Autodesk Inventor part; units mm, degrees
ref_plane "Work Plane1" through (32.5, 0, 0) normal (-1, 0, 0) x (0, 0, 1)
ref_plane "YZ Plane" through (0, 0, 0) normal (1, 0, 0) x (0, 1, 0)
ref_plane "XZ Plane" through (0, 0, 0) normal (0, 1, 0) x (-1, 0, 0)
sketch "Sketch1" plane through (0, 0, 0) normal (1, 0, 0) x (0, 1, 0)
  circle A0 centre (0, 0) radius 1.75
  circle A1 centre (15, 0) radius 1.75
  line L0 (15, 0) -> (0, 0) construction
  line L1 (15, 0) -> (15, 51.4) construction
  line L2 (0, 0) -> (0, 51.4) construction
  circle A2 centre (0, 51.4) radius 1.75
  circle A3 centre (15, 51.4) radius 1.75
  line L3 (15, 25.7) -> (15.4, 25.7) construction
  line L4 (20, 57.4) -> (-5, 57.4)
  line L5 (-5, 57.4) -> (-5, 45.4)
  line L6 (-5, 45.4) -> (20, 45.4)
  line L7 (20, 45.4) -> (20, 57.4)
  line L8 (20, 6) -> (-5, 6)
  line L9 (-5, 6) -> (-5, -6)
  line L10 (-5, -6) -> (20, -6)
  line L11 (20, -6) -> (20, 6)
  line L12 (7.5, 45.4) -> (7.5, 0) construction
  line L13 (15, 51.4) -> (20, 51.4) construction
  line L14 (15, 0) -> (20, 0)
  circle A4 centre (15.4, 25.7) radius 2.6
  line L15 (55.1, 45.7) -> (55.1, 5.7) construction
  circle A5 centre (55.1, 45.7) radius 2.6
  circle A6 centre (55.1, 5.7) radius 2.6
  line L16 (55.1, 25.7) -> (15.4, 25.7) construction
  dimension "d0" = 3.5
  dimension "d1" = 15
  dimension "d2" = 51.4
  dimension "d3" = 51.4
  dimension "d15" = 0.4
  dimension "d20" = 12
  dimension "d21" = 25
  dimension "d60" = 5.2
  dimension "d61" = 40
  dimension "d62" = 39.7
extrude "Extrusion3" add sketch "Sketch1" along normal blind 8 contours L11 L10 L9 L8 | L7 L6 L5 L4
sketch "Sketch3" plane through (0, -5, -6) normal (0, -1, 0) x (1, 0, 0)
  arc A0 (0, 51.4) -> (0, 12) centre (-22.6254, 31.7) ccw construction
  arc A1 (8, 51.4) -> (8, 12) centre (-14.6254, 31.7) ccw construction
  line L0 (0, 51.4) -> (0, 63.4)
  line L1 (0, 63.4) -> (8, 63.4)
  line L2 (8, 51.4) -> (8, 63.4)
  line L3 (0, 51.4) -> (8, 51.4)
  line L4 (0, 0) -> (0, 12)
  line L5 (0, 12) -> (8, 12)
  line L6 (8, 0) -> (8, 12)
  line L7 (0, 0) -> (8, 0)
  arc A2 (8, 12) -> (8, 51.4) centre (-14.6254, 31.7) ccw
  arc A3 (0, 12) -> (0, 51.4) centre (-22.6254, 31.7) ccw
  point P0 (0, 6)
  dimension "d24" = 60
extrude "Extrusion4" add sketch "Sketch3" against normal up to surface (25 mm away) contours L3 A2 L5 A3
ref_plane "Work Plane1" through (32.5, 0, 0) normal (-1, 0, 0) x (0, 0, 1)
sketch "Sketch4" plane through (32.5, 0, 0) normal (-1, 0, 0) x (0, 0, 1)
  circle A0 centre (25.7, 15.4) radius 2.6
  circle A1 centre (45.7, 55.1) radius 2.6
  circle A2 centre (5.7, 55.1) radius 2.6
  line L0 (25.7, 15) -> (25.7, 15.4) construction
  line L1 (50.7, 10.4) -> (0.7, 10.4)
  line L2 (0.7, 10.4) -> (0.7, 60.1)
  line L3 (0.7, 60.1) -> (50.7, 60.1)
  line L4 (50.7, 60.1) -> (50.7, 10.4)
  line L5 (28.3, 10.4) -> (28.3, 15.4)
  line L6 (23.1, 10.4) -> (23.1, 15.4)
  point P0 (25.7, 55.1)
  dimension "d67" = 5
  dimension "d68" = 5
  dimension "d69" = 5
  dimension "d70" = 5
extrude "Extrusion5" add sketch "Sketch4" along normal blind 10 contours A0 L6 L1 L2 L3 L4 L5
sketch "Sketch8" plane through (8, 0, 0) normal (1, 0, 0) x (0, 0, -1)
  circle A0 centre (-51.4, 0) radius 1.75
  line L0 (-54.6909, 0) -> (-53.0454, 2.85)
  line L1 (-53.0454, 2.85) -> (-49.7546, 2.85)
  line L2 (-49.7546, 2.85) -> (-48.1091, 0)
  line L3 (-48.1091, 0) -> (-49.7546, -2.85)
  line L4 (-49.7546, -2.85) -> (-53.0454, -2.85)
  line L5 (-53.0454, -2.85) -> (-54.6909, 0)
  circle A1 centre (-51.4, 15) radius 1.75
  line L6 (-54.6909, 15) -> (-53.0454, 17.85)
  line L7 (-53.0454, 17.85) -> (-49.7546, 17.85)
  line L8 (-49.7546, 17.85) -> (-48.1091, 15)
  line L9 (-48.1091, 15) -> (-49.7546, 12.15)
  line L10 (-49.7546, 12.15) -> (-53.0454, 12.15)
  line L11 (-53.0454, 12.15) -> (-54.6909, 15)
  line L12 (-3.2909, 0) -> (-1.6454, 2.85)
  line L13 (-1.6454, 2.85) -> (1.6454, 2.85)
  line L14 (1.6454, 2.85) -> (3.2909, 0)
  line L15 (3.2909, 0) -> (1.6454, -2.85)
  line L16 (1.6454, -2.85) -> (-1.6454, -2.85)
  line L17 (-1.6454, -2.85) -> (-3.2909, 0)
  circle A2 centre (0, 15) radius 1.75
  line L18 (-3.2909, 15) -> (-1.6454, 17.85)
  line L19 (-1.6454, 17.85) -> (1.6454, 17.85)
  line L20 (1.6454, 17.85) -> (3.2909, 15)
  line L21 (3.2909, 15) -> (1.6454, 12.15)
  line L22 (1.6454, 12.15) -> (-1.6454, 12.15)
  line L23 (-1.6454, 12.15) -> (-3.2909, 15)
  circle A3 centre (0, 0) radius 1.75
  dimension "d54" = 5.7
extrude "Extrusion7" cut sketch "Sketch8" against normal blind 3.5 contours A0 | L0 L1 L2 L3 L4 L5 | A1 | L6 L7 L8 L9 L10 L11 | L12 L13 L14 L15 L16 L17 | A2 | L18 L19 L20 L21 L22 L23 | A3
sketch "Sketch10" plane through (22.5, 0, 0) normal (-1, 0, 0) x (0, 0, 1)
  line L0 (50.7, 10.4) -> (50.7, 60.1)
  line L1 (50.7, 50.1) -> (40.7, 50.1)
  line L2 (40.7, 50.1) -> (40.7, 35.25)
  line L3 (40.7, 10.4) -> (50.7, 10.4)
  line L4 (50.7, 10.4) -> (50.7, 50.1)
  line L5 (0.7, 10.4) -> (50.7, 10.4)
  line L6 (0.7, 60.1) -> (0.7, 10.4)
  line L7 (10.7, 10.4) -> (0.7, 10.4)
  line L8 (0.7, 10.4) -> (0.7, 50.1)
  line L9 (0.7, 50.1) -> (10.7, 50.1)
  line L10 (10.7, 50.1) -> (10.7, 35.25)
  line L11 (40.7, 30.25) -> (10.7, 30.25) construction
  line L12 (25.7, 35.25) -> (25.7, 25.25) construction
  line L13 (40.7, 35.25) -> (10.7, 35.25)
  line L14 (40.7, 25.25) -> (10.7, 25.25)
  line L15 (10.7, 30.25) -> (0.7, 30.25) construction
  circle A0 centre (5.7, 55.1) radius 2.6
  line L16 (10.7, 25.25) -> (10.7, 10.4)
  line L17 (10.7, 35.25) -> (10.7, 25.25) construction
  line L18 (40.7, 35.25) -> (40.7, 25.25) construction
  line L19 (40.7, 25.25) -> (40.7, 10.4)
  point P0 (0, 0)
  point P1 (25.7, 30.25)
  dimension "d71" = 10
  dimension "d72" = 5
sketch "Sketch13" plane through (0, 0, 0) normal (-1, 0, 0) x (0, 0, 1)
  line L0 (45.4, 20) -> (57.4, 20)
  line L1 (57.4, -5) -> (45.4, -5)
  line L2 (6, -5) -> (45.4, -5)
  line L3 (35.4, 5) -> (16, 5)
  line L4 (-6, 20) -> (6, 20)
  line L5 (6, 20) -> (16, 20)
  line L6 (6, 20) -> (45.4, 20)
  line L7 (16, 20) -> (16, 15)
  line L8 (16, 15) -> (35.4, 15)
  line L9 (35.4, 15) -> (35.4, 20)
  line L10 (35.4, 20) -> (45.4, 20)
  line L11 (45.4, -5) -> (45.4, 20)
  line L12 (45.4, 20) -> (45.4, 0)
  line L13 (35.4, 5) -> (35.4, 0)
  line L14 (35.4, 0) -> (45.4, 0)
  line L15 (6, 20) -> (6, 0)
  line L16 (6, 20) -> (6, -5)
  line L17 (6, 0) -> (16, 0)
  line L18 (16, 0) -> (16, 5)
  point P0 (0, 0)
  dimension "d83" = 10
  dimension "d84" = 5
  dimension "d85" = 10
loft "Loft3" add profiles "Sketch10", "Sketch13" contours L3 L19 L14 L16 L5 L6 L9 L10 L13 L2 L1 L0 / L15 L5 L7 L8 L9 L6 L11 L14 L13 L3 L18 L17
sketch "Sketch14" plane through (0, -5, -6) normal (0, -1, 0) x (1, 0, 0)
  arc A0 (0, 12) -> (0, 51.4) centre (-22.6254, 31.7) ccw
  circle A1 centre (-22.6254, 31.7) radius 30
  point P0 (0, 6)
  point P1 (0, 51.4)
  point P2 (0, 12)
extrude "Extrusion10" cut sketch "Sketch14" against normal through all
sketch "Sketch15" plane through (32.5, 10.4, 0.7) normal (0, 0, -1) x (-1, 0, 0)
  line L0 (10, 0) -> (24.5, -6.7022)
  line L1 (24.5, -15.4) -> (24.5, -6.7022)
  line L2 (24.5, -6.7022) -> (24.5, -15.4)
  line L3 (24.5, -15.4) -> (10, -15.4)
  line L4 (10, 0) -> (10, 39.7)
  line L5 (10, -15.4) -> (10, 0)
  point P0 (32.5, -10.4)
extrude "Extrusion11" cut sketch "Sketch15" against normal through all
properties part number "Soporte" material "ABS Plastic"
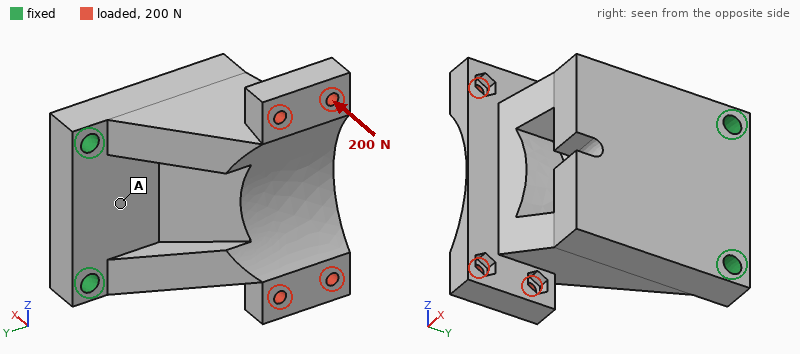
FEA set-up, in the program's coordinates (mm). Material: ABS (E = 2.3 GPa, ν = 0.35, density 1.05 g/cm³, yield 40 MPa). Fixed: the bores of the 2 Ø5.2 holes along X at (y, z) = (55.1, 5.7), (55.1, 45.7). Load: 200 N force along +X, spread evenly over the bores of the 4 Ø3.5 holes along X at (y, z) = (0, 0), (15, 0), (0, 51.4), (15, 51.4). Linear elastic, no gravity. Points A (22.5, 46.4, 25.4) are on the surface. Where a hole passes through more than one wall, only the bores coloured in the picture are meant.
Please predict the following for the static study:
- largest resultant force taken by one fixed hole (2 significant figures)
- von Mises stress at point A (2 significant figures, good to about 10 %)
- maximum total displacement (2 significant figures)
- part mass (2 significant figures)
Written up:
100 N
3.5 MPa
1.1 mm
49 g
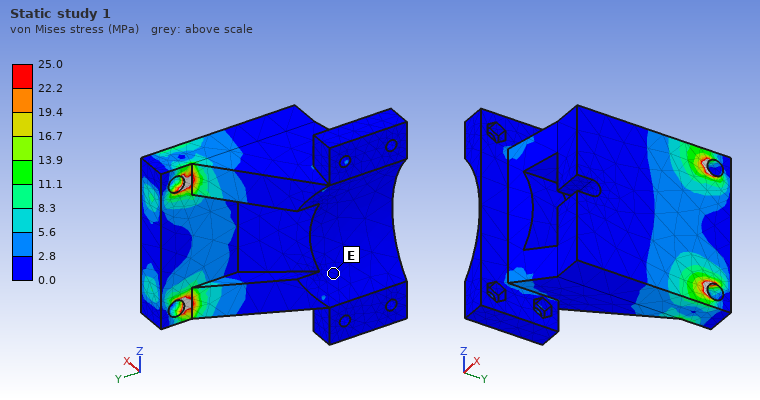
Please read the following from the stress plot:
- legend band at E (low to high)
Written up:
0.0 to 2.8 MPa
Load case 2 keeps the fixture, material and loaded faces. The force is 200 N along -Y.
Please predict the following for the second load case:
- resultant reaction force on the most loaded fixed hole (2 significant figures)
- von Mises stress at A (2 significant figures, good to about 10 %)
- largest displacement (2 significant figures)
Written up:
100 N
2.2 MPa
0.64 mm
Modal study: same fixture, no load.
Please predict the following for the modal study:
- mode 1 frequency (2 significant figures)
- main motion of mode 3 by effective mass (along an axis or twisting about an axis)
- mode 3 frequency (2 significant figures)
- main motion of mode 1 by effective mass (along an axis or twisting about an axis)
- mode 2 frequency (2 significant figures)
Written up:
550 Hz
along Z
2100 Hz
along X
1300 Hz
